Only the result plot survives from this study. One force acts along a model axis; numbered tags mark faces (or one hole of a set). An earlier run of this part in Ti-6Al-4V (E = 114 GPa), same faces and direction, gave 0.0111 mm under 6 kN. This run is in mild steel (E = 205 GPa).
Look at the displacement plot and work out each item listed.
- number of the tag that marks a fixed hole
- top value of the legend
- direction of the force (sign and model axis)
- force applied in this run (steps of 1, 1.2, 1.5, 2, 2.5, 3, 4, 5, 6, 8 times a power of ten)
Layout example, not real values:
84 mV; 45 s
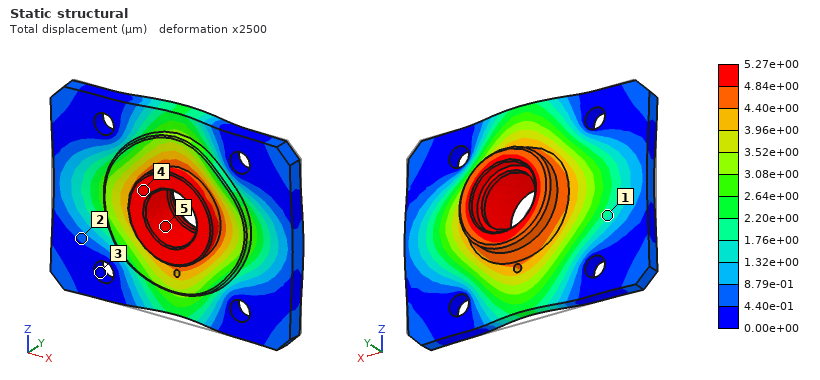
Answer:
3; 5.27e+00 µm; +Y; 5 kN
